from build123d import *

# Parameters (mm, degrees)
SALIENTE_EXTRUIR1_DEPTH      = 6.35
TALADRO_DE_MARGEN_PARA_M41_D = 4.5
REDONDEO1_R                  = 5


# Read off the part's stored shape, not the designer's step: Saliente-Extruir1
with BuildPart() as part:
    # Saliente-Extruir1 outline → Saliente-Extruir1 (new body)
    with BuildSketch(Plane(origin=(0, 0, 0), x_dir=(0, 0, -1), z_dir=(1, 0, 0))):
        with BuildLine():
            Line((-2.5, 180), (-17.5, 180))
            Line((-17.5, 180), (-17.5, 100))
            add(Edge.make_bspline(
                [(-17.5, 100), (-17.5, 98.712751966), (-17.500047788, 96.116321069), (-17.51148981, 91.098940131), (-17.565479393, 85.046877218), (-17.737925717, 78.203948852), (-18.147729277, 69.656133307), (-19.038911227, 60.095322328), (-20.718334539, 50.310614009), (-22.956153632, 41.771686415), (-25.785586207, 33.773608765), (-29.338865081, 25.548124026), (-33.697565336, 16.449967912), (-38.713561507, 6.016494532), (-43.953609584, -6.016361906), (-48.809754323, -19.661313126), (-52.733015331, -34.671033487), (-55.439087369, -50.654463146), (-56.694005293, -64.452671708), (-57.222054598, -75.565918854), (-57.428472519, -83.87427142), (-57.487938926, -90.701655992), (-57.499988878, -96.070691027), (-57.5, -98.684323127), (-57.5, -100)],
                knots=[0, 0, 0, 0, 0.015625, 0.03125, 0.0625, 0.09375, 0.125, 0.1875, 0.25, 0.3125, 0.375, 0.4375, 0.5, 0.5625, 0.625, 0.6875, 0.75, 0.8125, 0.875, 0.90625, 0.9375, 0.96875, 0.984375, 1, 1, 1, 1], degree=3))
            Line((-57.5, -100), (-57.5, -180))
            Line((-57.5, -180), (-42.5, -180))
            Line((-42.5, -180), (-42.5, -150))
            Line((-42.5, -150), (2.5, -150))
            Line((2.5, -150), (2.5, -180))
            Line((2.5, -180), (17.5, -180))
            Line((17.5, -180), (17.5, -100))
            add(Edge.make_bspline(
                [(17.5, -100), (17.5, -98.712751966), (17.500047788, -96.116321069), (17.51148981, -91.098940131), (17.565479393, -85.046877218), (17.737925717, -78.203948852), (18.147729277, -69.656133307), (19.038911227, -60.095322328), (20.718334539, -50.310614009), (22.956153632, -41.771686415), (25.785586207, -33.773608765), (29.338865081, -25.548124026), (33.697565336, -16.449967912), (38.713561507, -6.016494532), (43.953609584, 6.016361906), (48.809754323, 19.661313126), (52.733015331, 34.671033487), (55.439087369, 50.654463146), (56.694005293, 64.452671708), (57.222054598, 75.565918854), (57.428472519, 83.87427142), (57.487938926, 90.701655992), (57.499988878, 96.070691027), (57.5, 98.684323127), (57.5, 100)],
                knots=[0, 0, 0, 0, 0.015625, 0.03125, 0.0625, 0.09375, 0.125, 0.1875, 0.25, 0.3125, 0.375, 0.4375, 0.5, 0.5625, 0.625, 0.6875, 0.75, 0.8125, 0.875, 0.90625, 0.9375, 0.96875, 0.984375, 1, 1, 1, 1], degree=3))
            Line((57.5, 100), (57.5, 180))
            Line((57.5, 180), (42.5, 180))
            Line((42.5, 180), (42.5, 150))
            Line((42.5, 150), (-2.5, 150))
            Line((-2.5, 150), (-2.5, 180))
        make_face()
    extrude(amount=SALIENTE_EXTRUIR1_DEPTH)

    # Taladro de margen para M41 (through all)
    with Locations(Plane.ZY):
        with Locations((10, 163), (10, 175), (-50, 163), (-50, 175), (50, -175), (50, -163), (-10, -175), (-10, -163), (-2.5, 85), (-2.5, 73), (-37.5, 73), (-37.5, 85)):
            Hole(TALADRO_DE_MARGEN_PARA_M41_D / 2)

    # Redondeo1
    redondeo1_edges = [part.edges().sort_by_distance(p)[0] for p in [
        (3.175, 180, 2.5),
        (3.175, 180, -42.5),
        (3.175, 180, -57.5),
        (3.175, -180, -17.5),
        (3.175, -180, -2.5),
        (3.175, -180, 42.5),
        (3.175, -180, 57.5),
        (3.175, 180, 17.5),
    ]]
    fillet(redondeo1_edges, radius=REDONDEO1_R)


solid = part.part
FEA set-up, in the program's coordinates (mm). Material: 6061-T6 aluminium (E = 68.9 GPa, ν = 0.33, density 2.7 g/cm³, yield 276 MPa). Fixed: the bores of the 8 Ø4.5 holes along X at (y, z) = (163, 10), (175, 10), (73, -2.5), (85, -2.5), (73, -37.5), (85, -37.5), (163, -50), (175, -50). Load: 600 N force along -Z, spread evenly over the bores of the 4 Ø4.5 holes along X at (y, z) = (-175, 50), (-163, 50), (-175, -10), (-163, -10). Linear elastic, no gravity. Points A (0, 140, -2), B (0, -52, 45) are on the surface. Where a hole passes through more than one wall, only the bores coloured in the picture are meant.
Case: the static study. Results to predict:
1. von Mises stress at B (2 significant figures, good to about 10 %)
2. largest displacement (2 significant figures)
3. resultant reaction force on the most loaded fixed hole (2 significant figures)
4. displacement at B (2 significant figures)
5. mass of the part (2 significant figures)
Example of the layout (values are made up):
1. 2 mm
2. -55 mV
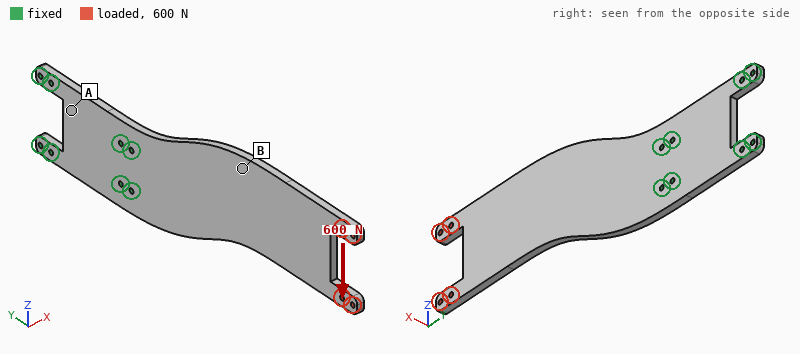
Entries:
1. 7.9 MPa
2. 0.30 mm
3. 2.3 kN
4. 0.11 mm
5. 420 g
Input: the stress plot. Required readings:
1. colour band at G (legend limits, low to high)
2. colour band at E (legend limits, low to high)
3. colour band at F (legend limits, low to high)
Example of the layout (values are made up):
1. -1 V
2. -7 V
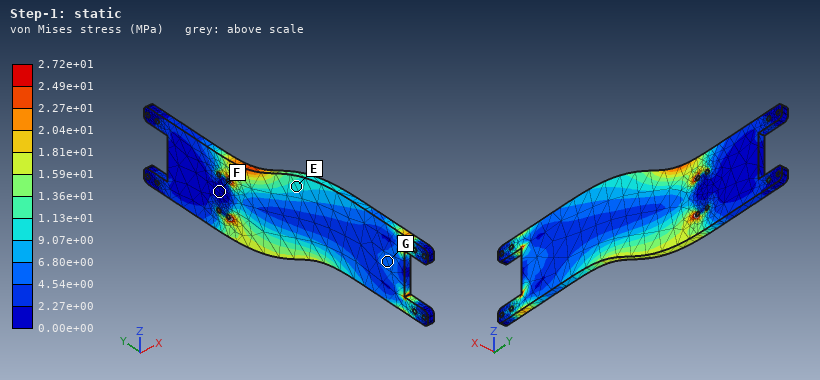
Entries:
1. 4.54e+00 to 6.80e+00 MPa
2. 9.07e+00 to 1.13e+01 MPa
3. 0.00e+00 to 2.27e+00 MPa
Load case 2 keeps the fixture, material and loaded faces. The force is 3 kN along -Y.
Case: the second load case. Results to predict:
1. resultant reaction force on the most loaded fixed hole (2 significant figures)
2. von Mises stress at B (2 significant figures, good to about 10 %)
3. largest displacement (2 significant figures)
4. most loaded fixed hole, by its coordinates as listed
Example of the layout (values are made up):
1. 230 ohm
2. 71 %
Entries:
1. 2.6 kN
2. 7.0 MPa
3. 0.19 mm
4. (73, -2.5)
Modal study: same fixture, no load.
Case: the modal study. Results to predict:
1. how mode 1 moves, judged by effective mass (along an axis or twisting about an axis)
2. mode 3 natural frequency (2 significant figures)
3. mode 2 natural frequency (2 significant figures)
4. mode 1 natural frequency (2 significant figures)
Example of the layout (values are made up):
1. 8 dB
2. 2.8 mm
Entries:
1. along X
2. 590 Hz
3. 500 Hz
4. 91 Hz
